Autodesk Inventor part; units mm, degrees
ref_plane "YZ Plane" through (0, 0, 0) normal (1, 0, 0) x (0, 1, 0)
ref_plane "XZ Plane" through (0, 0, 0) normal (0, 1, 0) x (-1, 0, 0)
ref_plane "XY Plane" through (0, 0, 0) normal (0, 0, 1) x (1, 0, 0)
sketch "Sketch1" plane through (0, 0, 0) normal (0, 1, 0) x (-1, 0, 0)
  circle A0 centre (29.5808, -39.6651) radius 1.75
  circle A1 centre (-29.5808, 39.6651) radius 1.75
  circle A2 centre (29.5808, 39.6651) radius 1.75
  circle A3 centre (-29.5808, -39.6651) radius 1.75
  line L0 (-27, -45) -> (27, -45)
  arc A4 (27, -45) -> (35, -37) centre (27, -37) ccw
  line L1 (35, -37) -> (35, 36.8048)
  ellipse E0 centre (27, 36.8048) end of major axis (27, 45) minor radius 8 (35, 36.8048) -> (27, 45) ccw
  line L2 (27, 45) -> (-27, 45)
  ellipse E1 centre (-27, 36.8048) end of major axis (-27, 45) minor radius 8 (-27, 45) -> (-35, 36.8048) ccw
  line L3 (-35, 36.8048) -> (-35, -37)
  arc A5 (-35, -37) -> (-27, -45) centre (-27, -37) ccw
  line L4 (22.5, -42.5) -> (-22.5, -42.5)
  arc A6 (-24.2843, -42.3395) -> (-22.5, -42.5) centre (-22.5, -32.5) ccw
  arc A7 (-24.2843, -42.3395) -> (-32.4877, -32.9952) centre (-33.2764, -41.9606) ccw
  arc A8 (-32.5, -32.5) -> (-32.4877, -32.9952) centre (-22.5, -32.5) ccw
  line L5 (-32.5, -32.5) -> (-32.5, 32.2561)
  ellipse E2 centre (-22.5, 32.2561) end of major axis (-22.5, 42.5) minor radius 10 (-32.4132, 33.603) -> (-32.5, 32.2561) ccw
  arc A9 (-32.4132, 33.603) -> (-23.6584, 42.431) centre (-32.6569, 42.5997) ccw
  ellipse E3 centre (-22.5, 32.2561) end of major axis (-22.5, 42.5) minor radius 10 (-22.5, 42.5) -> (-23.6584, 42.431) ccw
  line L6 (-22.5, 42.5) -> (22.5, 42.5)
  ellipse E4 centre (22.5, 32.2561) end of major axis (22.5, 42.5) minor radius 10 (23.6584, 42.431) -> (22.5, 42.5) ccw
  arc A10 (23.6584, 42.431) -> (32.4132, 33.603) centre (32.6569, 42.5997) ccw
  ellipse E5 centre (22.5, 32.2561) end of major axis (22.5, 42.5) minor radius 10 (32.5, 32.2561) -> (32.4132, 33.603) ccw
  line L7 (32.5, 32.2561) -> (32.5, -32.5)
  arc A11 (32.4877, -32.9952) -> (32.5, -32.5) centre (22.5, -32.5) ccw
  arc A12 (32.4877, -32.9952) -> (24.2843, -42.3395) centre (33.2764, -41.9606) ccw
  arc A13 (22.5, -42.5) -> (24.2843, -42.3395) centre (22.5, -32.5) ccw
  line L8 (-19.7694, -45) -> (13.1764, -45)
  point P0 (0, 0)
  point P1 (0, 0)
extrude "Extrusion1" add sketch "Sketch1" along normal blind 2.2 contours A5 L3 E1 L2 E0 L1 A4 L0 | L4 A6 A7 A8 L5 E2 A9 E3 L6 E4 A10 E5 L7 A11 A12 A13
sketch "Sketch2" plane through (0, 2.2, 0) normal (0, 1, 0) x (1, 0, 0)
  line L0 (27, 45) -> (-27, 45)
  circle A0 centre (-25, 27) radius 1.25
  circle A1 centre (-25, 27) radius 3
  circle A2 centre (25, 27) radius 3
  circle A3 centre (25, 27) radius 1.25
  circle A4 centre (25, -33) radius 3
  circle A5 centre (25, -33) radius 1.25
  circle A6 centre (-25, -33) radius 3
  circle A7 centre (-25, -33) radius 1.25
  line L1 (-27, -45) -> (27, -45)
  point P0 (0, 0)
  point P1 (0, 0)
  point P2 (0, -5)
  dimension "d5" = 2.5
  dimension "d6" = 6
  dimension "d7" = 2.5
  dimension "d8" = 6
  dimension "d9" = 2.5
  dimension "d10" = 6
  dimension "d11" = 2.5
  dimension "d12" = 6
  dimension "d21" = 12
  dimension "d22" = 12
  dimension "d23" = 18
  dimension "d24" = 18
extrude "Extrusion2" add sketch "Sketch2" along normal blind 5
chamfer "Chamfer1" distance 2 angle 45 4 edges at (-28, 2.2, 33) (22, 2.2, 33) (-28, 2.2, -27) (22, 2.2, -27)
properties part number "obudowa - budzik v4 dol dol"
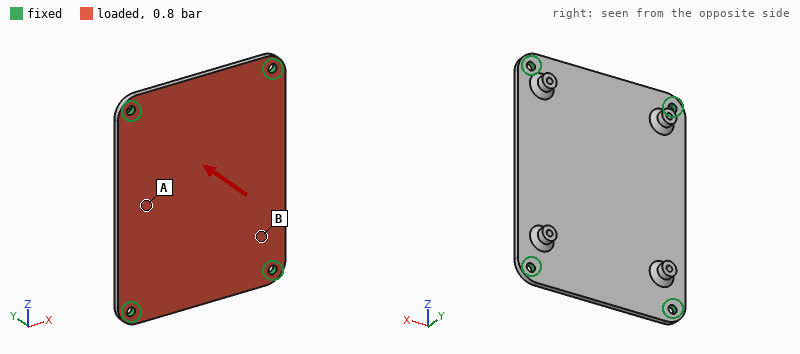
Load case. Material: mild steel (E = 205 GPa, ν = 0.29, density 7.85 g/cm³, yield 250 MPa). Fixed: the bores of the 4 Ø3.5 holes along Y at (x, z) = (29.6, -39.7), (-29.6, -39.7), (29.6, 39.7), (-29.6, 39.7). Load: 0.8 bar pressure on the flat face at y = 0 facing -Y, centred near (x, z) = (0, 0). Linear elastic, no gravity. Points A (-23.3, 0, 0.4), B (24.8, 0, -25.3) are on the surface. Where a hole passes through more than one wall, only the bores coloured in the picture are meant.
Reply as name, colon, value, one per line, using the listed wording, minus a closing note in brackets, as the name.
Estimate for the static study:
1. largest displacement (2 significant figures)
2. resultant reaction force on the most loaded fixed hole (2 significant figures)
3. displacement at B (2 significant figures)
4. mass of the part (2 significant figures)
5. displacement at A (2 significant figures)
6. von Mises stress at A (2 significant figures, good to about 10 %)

largest displacement: 75 µm
resultant reaction force on the most loaded fixed hole: 130 N
displacement at B: 28 µm
mass of the part: 110 g
displacement at A: 64 µm
von Mises stress at A: 29 MPa
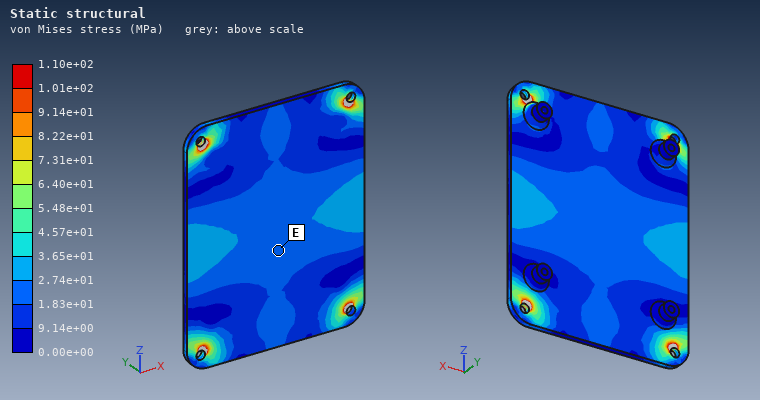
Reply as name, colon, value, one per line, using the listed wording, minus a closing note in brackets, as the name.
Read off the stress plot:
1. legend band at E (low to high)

legend band at E: 1.83e+01 to 2.74e+01 MPa
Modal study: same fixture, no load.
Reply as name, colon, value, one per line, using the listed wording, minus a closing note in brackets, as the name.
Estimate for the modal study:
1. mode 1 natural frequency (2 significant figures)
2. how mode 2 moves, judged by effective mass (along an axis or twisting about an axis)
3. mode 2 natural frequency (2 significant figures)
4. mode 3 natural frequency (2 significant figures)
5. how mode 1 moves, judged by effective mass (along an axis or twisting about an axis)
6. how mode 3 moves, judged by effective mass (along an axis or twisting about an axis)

mode 1 natural frequency: 1500 Hz
how mode 2 moves, judged by effective mass: twisting about Z
mode 2 natural frequency: 2400 Hz
mode 3 natural frequency: 3300 Hz
how mode 1 moves, judged by effective mass: along Y
how mode 3 moves, judged by effective mass: twisting about X
